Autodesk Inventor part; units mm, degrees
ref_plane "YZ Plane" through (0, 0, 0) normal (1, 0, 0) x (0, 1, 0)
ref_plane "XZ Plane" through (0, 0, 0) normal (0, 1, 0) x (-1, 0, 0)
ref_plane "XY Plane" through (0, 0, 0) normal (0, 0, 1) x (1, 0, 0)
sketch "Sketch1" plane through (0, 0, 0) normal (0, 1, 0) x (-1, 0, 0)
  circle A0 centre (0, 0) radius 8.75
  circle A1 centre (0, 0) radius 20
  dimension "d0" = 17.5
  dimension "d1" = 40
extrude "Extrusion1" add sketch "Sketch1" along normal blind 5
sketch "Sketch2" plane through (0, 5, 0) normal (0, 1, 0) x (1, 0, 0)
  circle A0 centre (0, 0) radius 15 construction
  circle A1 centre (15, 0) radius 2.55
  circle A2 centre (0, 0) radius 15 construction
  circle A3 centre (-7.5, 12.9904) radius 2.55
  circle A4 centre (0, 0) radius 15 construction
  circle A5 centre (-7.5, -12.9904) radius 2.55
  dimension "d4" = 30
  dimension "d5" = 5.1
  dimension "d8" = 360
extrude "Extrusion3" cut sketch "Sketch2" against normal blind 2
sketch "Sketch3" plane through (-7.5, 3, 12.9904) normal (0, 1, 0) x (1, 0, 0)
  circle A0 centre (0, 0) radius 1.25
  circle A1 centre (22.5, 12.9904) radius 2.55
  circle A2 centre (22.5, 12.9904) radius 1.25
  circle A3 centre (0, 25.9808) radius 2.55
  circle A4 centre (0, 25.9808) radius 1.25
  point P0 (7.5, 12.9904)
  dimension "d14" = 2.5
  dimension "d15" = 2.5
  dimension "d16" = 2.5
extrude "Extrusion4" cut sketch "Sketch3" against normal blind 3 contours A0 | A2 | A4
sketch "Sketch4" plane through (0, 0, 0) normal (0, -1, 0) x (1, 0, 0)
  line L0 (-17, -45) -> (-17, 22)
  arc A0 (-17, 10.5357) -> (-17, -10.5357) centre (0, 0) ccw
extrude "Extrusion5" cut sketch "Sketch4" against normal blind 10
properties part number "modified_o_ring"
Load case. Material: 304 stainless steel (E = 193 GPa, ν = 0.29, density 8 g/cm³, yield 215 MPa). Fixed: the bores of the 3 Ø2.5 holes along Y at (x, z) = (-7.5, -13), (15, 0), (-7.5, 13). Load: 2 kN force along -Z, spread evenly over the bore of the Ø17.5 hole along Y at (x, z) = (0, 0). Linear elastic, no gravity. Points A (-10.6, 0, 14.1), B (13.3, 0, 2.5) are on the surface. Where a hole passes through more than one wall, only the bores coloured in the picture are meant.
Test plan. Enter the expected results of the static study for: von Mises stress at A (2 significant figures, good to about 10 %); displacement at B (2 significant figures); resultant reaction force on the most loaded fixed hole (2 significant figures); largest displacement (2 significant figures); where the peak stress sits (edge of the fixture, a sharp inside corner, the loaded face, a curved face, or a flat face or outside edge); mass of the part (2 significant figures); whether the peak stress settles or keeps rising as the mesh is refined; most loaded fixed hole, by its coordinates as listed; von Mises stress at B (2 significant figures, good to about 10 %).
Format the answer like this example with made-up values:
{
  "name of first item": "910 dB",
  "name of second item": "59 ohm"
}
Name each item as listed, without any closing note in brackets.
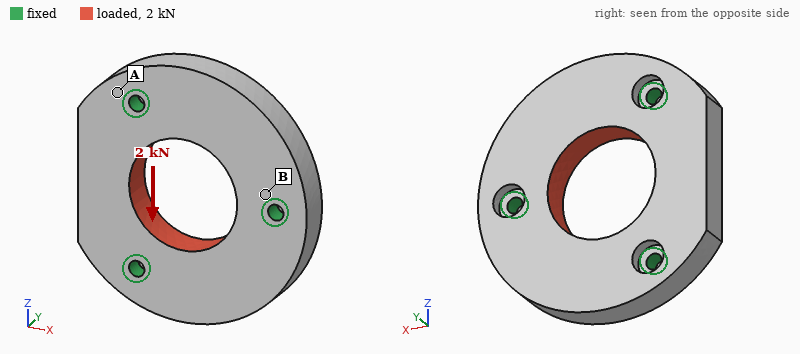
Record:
{
  "von Mises stress at A": "9.4 MPa",
  "displacement at B": "0.32 µm",
  "resultant reaction force on the most loaded fixed hole": "770 N",
  "largest displacement": "2.1 µm",
  "where the peak stress sits": "edge of the fixture",
  "mass of the part": "38 g",
  "whether the peak stress settles or keeps rising as the mesh is refined": "keeps rising",
  "most loaded fixed hole, by its coordinates as listed": "(15, 0)",
  "von Mises stress at B": "21 MPa"
}
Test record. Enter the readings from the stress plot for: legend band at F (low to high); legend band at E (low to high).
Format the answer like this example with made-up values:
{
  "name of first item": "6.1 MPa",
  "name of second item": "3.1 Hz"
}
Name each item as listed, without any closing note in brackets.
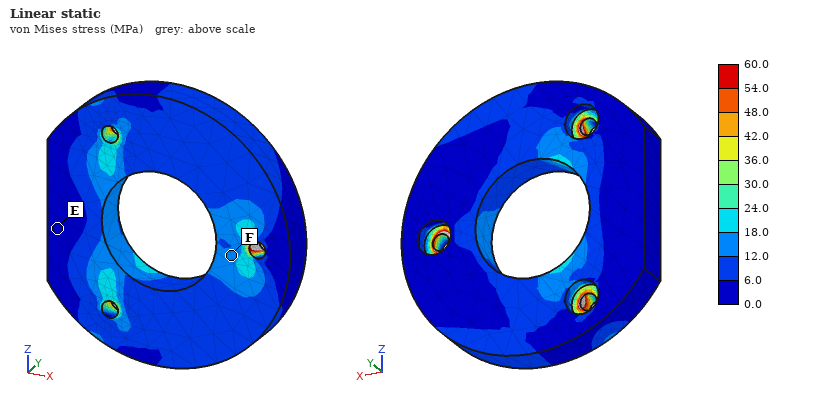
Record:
{
  "legend band at F": "12.0 to 18.0 MPa",
  "legend band at E": "0.0 to 6.0 MPa"
}
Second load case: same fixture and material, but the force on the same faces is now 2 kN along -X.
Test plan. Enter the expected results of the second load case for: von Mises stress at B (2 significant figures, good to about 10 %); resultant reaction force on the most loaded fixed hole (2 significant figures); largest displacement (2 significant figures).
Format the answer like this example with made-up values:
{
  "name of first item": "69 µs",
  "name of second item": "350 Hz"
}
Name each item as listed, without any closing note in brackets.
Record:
{
  "von Mises stress at B": "12 MPa",
  "resultant reaction force on the most loaded fixed hole": "730 N",
  "largest displacement": "2.5 µm"
}
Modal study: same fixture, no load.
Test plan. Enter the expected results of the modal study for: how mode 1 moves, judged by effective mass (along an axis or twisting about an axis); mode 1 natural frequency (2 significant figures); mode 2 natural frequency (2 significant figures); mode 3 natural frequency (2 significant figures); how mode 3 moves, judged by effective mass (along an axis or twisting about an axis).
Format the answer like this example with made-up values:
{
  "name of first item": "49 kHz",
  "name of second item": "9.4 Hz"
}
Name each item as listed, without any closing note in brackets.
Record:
{
  "how mode 1 moves, judged by effective mass": "twisting about X",
  "mode 1 natural frequency": "13 kHz",
  "mode 2 natural frequency": "15 kHz",
  "mode 3 natural frequency": "20 kHz",
  "how mode 3 moves, judged by effective mass": "along Y"
}
